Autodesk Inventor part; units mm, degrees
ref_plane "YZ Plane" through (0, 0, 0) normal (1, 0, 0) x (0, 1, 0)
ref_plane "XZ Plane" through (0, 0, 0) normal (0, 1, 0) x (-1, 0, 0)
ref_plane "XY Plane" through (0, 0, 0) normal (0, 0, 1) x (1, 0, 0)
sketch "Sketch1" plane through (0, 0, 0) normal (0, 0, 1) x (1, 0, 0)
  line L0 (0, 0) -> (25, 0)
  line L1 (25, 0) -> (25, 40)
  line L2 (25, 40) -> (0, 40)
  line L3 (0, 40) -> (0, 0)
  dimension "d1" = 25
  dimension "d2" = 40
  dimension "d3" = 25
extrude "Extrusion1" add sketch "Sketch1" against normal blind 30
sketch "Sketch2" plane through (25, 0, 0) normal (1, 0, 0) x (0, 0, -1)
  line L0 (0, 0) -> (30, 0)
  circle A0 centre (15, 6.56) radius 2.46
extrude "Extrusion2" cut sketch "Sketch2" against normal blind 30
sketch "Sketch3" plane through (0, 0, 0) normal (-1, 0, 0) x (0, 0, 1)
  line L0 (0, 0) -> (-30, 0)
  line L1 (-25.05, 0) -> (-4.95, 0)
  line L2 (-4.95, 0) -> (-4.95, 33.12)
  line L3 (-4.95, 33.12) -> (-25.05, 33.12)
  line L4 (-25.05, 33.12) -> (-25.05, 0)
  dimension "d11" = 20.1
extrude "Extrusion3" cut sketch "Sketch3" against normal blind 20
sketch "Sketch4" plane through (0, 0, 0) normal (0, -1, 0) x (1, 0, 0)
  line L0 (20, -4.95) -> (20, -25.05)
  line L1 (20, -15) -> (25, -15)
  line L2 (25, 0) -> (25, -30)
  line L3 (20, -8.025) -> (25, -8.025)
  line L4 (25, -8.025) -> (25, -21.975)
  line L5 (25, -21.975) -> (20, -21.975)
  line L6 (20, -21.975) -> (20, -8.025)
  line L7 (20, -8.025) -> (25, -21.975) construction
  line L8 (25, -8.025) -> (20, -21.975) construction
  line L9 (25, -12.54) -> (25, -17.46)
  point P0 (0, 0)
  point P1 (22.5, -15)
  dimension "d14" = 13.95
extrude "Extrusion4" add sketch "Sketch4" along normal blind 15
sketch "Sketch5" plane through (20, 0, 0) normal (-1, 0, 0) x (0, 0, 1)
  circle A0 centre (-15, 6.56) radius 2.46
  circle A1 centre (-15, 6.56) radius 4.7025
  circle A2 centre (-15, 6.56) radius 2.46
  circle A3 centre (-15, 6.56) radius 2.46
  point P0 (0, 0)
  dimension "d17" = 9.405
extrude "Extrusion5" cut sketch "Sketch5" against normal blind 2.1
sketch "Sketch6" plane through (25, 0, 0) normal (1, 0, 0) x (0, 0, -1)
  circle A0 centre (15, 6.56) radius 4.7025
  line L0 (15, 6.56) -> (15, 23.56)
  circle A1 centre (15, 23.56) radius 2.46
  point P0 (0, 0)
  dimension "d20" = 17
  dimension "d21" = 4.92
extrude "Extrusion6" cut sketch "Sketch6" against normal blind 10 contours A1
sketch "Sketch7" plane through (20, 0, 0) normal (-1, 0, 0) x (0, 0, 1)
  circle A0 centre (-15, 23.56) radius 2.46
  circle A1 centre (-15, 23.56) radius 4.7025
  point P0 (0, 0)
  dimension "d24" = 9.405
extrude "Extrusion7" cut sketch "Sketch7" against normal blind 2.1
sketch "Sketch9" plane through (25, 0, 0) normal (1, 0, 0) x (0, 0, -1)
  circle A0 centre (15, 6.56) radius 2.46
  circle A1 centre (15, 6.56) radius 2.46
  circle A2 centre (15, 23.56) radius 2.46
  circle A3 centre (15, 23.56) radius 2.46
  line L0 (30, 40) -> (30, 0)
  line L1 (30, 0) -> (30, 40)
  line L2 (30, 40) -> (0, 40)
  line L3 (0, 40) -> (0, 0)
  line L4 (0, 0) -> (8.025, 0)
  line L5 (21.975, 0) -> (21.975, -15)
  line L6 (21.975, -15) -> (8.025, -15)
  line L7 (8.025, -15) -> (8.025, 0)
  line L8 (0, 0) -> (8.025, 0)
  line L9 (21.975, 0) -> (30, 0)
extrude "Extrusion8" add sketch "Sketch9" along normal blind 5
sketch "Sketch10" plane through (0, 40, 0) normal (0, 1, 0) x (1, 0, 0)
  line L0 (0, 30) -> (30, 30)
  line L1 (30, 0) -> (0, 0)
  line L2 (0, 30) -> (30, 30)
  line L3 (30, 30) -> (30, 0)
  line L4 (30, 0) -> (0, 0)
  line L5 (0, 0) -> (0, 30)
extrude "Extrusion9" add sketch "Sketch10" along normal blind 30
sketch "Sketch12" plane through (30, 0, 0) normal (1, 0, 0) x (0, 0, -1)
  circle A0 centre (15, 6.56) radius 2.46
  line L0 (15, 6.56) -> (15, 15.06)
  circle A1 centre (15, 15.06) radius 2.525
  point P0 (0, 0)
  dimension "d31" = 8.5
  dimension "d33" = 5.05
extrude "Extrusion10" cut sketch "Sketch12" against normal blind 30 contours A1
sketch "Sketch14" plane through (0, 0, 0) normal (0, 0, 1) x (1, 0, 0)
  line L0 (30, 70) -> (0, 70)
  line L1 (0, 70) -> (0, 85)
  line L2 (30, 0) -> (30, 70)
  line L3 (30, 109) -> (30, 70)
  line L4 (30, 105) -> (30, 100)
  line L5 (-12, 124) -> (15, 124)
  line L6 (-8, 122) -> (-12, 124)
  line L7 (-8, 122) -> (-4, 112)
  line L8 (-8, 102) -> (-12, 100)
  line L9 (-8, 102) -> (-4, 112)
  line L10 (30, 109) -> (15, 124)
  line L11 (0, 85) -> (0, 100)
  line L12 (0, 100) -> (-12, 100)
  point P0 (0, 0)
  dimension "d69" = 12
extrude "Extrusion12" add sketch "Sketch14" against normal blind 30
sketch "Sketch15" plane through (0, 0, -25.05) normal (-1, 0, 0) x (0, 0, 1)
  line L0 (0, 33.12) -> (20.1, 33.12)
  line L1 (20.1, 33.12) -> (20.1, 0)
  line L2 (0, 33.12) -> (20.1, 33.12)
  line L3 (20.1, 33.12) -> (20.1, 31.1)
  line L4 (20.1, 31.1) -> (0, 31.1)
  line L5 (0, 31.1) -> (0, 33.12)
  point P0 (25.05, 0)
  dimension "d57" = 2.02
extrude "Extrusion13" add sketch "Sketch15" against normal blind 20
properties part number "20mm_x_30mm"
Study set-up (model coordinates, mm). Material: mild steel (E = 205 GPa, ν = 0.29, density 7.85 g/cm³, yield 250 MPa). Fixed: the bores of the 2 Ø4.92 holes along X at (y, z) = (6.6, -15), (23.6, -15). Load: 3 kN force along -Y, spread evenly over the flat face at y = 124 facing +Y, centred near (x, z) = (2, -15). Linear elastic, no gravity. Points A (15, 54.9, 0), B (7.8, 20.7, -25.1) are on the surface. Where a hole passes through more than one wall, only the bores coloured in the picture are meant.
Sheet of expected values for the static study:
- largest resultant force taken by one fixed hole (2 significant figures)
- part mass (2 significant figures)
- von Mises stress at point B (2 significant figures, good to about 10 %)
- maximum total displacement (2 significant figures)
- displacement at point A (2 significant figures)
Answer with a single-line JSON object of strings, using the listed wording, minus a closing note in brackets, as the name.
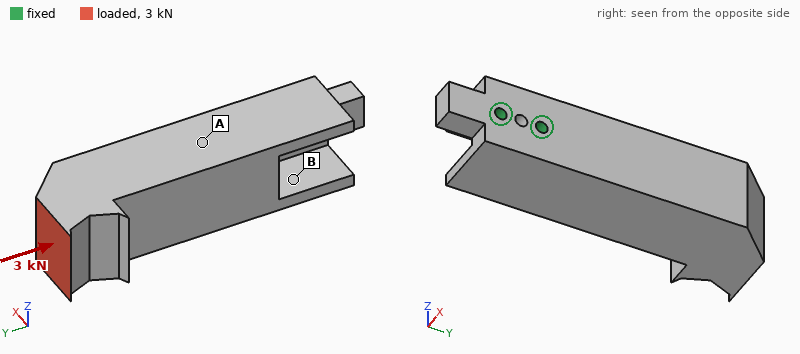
{"largest resultant force taken by one fixed hole": "3.4 kN", "part mass": "800 g", "von Mises stress at point B": "22 MPa", "maximum total displacement": "75 µm", "displacement at point A": "18 µm"}
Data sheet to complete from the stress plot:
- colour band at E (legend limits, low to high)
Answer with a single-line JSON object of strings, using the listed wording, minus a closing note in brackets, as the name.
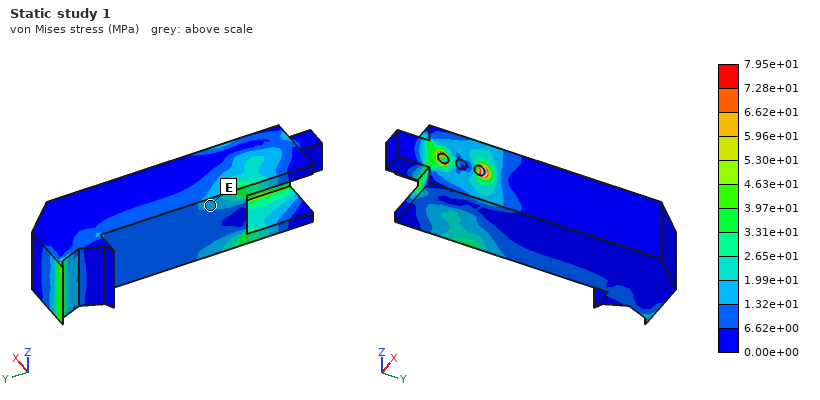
{"colour band at E": "1.32e+01 to 1.99e+01 MPa"}
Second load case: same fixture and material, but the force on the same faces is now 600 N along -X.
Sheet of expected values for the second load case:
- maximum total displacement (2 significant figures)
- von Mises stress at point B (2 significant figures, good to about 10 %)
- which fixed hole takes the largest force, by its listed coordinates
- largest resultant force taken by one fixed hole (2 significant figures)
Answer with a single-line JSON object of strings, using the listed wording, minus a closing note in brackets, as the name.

{"maximum total displacement": "62 µm", "von Mises stress at point B": "17 MPa", "which fixed hole takes the largest force, by its listed coordinates": "(23.6, -15)", "largest resultant force taken by one fixed hole": "3.0 kN"}
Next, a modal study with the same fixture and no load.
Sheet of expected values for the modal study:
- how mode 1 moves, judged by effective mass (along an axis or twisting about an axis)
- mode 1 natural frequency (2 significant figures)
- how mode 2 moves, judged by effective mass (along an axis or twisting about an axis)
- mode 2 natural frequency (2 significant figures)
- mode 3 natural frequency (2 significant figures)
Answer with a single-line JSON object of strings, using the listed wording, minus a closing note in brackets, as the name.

{"how mode 1 moves, judged by effective mass": "along X", "mode 1 natural frequency": "1000 Hz", "how mode 2 moves, judged by effective mass": "along Z", "mode 2 natural frequency": "1200 Hz", "mode 3 natural frequency": "3200 Hz"}
